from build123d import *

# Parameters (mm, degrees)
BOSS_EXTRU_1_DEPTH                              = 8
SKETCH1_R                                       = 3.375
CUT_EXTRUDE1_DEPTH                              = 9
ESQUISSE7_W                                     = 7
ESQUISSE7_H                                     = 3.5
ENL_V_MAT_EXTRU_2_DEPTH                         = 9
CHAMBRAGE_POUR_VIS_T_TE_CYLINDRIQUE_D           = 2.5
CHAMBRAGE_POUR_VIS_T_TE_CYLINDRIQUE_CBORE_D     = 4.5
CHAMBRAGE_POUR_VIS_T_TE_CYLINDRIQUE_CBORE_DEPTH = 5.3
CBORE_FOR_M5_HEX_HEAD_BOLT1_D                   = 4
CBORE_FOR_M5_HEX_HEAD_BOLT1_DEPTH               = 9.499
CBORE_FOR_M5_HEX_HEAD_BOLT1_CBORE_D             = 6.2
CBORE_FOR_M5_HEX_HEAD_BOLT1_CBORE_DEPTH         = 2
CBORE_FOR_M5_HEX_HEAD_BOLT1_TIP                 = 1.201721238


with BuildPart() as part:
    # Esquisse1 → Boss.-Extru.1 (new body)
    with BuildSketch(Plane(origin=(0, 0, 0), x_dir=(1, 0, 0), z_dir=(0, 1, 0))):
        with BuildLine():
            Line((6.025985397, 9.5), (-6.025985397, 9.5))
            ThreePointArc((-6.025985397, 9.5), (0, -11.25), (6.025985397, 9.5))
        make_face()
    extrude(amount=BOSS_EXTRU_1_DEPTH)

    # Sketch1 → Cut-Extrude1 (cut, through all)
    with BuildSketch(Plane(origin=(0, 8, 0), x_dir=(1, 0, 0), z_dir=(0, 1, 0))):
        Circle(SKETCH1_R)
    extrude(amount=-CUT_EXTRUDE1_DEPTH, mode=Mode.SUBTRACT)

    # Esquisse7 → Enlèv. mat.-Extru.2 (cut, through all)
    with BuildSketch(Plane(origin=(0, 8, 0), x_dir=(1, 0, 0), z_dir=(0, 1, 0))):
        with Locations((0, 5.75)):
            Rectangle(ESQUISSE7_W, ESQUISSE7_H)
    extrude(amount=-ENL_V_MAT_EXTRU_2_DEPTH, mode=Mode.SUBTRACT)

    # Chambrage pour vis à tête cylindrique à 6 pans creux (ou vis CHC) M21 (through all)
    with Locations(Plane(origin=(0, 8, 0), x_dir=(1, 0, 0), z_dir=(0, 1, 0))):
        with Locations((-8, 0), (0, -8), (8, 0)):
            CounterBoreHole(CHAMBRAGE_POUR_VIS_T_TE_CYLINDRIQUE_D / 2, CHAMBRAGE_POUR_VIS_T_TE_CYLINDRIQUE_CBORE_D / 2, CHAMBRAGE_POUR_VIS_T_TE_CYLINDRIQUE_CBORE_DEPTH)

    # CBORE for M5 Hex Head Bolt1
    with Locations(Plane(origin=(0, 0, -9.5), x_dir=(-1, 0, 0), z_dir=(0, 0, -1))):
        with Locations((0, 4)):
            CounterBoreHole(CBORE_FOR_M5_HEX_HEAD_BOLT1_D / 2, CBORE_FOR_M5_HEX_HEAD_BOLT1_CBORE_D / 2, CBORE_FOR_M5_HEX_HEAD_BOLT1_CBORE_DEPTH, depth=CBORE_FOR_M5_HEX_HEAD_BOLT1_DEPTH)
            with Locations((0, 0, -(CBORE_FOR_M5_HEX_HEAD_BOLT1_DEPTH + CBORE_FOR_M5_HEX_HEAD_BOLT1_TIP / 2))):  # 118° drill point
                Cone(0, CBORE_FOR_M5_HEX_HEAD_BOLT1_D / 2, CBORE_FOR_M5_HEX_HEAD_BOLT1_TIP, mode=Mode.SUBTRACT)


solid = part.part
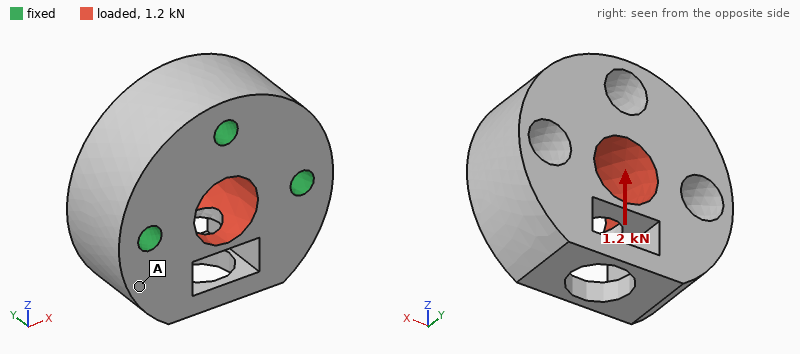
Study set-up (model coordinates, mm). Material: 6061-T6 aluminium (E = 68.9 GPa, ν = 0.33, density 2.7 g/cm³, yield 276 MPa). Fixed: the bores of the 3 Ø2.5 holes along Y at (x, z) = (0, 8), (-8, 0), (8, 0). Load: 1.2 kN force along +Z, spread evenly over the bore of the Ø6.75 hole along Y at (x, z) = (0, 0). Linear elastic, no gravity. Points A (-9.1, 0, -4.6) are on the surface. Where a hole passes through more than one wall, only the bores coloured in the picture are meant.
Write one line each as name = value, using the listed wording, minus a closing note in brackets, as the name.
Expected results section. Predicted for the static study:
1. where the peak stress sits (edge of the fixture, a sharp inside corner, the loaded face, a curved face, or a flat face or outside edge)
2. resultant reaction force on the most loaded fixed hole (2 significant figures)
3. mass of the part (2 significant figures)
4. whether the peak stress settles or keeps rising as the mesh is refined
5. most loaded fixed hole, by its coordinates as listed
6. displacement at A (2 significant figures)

where the peak stress sits = edge of the fixture
resultant reaction force on the most loaded fixed hole = 530 N
mass of the part = 6.0 g
whether the peak stress settles or keeps rising as the mesh is refined = keeps rising
most loaded fixed hole, by its coordinates as listed = (0, 8)
displacement at A = 2.0 µm
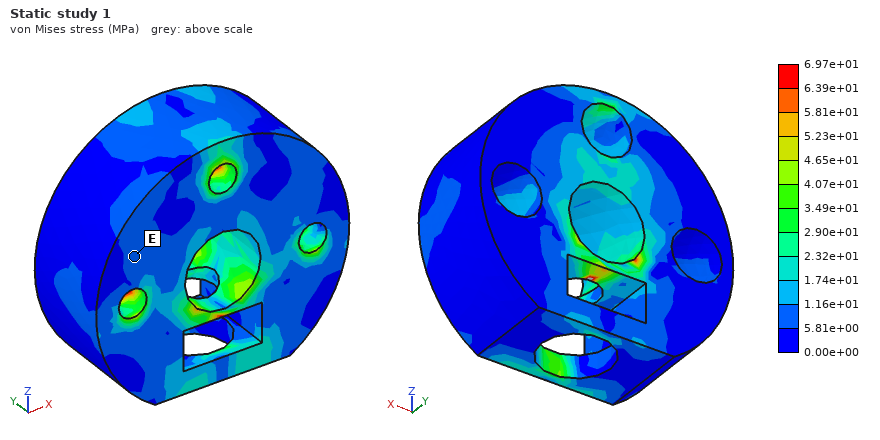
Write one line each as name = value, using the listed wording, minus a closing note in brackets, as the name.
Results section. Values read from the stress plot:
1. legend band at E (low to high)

legend band at E = 5.81e+00 to 1.16e+01 MPa
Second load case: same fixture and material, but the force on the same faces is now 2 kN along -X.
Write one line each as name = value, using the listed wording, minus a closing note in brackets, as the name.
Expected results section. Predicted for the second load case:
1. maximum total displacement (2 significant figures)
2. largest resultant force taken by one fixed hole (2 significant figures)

maximum total displacement = 7.1 µm
largest resultant force taken by one fixed hole = 830 N
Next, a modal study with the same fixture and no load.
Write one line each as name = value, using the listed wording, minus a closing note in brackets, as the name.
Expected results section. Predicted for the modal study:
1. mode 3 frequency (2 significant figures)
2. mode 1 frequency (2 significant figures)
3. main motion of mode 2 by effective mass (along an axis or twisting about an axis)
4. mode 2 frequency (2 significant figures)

mode 3 frequency = 41 kHz
mode 1 frequency = 28 kHz
main motion of mode 2 by effective mass = along X
mode 2 frequency = 34 kHz
